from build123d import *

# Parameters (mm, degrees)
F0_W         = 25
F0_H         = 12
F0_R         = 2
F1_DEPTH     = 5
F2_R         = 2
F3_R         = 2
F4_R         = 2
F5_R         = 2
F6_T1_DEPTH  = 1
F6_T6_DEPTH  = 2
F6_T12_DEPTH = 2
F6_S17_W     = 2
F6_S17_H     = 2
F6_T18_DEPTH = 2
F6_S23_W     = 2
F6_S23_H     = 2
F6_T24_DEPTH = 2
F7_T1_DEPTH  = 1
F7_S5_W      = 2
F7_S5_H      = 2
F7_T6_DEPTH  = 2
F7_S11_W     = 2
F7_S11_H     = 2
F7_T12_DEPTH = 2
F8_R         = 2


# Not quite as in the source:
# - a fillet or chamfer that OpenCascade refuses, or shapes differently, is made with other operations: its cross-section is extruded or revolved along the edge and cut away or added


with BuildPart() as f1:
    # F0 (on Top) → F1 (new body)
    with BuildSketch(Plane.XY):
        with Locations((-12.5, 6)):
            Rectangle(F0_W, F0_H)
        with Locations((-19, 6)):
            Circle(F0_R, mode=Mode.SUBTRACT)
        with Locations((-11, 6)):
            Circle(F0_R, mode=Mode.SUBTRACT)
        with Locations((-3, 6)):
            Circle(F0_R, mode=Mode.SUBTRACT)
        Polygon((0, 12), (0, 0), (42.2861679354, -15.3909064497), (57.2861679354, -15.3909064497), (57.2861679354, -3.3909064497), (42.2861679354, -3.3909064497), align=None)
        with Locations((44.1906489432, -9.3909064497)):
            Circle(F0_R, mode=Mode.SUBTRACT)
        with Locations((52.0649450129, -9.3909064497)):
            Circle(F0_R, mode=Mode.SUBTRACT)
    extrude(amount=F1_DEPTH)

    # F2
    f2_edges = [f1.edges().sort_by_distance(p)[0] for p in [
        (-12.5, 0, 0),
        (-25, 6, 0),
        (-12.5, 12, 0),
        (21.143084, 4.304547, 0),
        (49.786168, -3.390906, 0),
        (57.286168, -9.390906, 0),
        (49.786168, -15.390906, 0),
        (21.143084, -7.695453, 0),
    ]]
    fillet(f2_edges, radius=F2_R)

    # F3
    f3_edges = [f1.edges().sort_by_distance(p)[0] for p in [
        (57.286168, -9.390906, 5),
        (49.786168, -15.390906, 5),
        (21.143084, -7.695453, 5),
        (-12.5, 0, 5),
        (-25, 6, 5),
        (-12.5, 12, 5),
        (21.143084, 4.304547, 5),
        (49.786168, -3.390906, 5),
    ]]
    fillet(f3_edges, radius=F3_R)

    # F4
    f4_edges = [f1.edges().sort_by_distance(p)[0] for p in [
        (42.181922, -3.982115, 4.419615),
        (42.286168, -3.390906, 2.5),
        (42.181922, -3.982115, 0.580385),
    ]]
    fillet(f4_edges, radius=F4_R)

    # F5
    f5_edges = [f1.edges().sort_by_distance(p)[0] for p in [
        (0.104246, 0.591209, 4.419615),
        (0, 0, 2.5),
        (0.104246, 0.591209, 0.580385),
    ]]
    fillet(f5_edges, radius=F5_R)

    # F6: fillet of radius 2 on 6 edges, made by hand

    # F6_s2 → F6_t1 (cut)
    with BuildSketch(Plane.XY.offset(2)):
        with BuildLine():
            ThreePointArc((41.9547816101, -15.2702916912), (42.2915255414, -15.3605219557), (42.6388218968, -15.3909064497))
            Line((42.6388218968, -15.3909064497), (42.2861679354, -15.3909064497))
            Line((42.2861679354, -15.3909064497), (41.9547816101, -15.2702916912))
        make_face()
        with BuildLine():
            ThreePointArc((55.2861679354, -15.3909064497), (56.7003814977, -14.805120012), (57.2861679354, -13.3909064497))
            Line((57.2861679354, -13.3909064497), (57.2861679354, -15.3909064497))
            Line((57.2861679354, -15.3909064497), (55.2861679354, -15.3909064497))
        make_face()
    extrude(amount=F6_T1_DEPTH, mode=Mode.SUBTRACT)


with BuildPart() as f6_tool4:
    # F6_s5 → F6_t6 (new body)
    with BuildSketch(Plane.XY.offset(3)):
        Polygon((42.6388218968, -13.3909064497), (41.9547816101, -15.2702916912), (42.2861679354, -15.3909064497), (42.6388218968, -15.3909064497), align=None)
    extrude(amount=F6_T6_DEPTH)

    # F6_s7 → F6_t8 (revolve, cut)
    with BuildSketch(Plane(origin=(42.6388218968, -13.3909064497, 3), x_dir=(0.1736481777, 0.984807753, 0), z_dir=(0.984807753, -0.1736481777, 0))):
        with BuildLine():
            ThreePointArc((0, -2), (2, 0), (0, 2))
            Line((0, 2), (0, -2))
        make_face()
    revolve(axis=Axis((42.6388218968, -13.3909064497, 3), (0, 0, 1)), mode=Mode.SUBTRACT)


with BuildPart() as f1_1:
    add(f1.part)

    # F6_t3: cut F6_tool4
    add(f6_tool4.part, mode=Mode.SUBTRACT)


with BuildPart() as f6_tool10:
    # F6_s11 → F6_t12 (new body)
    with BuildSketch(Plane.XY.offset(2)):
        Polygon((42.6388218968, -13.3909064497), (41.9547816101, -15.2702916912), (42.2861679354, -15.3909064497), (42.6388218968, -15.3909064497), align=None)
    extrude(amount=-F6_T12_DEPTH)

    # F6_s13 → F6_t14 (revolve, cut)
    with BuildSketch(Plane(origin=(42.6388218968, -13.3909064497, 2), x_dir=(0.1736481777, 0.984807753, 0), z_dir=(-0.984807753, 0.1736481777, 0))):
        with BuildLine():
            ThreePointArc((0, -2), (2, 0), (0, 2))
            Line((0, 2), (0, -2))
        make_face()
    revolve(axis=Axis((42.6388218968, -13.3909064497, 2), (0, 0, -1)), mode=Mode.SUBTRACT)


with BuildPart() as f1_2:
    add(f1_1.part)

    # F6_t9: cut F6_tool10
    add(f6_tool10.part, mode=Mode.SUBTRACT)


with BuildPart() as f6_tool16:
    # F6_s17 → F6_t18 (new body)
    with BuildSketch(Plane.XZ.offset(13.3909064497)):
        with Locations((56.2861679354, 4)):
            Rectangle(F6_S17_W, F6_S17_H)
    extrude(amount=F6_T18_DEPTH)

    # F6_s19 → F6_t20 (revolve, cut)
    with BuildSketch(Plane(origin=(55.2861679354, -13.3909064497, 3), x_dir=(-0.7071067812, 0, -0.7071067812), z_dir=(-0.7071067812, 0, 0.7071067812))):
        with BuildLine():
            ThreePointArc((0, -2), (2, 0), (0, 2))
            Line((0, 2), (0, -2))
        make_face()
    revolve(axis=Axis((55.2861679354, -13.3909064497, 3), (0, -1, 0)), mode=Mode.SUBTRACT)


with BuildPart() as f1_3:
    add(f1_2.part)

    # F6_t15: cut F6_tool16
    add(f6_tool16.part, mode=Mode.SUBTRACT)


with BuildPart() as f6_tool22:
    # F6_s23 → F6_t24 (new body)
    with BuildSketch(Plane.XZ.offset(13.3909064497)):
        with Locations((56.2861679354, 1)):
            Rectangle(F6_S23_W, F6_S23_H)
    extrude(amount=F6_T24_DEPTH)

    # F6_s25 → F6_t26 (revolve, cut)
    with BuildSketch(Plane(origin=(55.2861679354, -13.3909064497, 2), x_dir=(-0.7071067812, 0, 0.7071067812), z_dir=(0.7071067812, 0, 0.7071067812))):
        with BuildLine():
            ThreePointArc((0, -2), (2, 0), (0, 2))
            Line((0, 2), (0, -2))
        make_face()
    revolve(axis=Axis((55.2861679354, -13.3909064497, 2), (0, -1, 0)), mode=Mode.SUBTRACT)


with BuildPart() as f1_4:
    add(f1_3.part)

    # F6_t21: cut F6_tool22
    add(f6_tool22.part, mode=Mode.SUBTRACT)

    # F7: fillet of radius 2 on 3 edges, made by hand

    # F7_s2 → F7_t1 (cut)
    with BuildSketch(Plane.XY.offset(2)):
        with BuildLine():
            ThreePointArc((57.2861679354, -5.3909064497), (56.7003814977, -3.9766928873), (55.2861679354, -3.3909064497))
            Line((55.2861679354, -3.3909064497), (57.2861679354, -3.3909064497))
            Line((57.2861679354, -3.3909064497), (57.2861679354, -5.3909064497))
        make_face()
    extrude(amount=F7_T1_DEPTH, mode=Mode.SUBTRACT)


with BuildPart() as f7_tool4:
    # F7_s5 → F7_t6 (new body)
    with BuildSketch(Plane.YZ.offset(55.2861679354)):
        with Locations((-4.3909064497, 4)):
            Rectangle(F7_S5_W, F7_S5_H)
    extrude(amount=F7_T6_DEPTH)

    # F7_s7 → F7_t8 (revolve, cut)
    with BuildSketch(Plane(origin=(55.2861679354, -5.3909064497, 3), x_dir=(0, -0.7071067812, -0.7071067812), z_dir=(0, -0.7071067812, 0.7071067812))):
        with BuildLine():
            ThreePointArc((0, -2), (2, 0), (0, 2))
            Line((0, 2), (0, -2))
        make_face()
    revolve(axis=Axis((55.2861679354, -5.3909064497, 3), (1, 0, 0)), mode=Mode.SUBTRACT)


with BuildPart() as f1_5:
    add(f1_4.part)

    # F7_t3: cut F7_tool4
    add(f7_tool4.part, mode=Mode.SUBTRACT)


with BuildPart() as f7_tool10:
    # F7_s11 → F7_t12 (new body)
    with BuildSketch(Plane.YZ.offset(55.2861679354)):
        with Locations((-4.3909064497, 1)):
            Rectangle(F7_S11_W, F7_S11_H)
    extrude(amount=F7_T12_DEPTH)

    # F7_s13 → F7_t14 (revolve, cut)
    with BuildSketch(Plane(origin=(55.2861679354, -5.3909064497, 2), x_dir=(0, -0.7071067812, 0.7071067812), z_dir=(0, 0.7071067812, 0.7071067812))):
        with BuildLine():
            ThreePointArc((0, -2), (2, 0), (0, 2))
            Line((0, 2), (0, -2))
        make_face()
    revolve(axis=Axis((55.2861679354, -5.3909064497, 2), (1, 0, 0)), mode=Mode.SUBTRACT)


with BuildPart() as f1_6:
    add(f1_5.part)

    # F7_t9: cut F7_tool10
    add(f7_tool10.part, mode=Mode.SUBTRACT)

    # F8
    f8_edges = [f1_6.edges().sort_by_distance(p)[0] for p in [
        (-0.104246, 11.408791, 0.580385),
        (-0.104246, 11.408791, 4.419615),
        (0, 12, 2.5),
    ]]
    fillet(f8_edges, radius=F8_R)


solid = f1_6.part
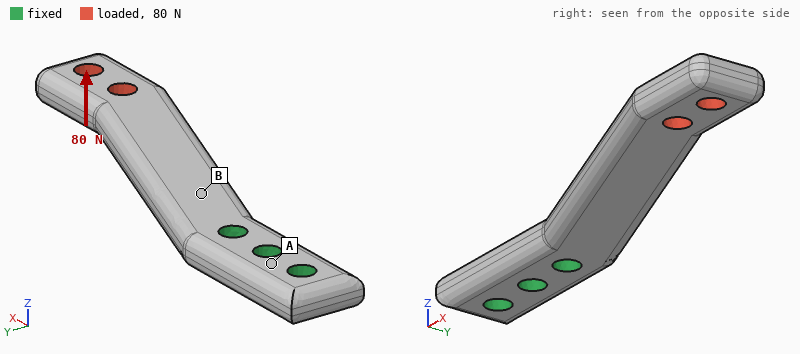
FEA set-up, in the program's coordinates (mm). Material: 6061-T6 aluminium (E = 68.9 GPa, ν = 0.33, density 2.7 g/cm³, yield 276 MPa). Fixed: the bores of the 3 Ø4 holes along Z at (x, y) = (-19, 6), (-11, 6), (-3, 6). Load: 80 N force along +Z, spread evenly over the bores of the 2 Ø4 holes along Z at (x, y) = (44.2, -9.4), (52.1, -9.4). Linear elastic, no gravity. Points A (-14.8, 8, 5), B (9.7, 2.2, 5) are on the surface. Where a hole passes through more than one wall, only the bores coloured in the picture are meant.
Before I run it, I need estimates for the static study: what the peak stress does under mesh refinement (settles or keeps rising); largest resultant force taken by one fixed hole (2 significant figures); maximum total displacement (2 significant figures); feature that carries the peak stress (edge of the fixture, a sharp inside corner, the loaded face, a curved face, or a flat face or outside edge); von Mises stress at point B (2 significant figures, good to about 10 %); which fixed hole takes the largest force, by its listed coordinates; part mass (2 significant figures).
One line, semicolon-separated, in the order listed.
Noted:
keeps rising; 150 N; 0.70 mm; edge of the fixture; 78 MPa; (-3, 6); 12 g
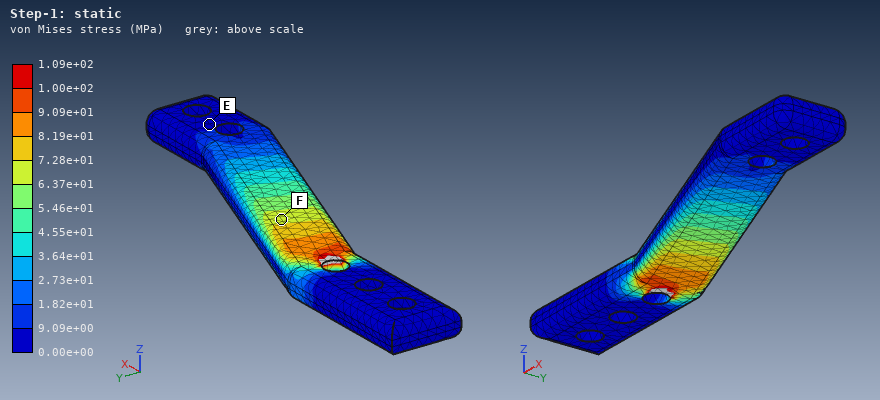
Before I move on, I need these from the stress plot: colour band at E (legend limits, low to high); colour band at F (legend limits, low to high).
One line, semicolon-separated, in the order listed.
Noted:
0.00e+00 to 9.09e+00 MPa; 6.37e+01 to 7.28e+01 MPa
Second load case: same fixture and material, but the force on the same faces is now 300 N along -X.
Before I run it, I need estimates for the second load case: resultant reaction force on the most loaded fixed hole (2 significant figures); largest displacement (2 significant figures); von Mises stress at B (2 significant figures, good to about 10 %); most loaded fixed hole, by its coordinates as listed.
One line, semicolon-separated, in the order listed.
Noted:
320 N; 0.18 mm; 8.9 MPa; (-3, 6)
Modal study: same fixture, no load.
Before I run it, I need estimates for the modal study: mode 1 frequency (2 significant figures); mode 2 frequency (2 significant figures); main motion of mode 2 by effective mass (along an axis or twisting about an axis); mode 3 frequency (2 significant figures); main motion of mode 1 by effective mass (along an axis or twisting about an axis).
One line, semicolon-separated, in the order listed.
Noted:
1100 Hz; 2200 Hz; along Y; 6300 Hz; along Z
